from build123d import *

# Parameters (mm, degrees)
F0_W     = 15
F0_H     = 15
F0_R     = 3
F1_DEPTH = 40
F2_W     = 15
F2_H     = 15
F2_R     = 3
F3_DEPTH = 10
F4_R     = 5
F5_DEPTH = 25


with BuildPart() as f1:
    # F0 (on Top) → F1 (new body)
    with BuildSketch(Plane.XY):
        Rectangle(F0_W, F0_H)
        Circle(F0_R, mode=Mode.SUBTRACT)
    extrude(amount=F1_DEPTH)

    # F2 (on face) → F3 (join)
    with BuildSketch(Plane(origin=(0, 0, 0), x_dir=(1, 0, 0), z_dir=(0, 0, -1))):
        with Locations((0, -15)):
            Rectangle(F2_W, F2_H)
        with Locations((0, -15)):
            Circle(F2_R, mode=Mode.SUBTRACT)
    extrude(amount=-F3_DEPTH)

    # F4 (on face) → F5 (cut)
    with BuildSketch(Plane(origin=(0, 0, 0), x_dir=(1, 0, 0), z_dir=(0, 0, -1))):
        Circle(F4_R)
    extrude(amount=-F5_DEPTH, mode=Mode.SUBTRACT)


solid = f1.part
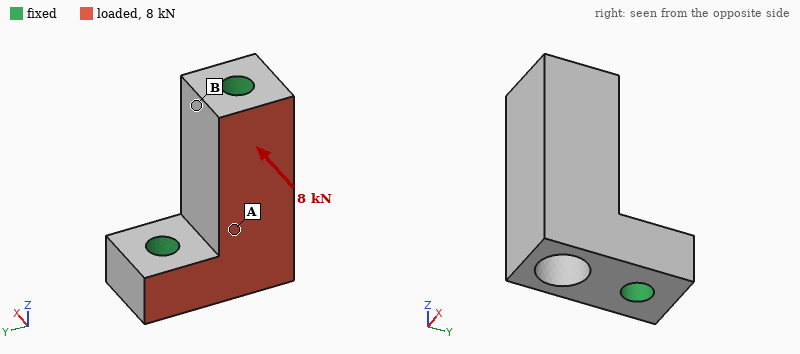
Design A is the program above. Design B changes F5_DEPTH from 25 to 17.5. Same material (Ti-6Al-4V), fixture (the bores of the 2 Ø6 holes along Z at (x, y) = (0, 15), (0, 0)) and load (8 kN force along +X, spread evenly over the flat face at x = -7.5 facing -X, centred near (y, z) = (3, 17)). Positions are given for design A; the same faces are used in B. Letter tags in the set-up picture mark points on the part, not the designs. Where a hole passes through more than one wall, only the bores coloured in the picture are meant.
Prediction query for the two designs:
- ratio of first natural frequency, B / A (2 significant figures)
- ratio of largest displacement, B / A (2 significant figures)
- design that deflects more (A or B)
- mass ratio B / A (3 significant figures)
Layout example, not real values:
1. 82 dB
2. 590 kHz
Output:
1. 1.3
2. 0.62
3. A
4. 1.04
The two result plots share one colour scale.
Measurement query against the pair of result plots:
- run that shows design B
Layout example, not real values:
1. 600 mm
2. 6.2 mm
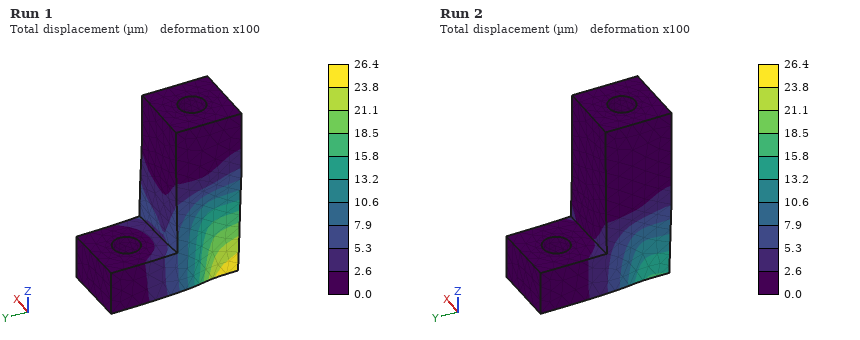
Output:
1. Run 2
